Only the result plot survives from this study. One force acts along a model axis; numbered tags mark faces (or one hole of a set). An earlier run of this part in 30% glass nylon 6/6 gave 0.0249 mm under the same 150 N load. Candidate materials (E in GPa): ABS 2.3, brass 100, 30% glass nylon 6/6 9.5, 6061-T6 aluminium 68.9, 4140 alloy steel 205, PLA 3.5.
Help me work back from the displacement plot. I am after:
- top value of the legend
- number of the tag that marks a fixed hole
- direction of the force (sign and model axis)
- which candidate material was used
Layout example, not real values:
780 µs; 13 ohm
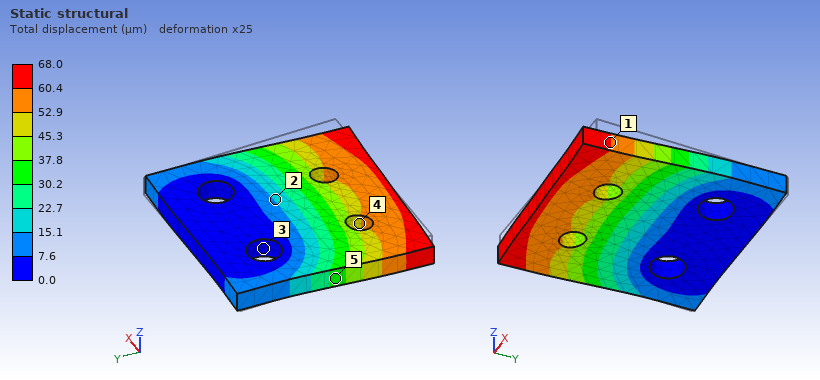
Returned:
68.0 µm; 3; -X; PLA
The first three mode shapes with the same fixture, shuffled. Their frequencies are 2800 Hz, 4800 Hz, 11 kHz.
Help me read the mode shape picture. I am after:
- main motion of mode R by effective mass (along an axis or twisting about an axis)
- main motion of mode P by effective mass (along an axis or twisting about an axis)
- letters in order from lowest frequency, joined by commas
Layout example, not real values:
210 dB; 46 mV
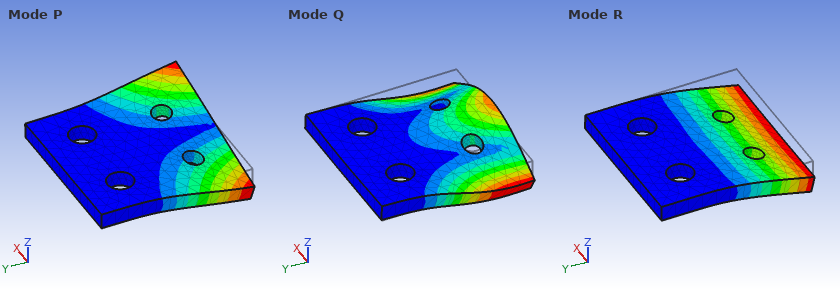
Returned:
along Z; twisting about Y; R, P, Q
